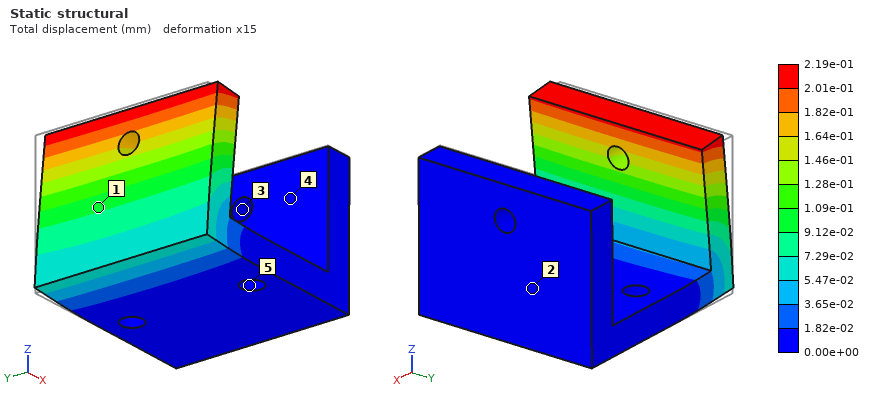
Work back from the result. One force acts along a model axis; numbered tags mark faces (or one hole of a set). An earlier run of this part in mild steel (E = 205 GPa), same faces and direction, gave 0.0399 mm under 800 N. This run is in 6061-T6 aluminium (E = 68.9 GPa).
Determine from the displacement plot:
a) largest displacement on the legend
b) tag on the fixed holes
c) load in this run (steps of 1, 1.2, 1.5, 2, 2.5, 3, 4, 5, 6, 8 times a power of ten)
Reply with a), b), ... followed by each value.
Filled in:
a) 2.19e-01 mm
b) 5
c) 1.5 kN
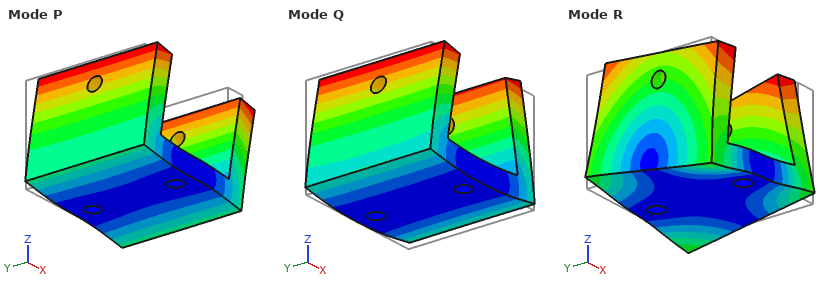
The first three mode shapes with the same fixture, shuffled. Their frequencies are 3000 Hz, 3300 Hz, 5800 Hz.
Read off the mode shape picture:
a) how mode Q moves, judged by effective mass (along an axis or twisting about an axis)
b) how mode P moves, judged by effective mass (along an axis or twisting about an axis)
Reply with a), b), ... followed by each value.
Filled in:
a) along Z
b) along X
